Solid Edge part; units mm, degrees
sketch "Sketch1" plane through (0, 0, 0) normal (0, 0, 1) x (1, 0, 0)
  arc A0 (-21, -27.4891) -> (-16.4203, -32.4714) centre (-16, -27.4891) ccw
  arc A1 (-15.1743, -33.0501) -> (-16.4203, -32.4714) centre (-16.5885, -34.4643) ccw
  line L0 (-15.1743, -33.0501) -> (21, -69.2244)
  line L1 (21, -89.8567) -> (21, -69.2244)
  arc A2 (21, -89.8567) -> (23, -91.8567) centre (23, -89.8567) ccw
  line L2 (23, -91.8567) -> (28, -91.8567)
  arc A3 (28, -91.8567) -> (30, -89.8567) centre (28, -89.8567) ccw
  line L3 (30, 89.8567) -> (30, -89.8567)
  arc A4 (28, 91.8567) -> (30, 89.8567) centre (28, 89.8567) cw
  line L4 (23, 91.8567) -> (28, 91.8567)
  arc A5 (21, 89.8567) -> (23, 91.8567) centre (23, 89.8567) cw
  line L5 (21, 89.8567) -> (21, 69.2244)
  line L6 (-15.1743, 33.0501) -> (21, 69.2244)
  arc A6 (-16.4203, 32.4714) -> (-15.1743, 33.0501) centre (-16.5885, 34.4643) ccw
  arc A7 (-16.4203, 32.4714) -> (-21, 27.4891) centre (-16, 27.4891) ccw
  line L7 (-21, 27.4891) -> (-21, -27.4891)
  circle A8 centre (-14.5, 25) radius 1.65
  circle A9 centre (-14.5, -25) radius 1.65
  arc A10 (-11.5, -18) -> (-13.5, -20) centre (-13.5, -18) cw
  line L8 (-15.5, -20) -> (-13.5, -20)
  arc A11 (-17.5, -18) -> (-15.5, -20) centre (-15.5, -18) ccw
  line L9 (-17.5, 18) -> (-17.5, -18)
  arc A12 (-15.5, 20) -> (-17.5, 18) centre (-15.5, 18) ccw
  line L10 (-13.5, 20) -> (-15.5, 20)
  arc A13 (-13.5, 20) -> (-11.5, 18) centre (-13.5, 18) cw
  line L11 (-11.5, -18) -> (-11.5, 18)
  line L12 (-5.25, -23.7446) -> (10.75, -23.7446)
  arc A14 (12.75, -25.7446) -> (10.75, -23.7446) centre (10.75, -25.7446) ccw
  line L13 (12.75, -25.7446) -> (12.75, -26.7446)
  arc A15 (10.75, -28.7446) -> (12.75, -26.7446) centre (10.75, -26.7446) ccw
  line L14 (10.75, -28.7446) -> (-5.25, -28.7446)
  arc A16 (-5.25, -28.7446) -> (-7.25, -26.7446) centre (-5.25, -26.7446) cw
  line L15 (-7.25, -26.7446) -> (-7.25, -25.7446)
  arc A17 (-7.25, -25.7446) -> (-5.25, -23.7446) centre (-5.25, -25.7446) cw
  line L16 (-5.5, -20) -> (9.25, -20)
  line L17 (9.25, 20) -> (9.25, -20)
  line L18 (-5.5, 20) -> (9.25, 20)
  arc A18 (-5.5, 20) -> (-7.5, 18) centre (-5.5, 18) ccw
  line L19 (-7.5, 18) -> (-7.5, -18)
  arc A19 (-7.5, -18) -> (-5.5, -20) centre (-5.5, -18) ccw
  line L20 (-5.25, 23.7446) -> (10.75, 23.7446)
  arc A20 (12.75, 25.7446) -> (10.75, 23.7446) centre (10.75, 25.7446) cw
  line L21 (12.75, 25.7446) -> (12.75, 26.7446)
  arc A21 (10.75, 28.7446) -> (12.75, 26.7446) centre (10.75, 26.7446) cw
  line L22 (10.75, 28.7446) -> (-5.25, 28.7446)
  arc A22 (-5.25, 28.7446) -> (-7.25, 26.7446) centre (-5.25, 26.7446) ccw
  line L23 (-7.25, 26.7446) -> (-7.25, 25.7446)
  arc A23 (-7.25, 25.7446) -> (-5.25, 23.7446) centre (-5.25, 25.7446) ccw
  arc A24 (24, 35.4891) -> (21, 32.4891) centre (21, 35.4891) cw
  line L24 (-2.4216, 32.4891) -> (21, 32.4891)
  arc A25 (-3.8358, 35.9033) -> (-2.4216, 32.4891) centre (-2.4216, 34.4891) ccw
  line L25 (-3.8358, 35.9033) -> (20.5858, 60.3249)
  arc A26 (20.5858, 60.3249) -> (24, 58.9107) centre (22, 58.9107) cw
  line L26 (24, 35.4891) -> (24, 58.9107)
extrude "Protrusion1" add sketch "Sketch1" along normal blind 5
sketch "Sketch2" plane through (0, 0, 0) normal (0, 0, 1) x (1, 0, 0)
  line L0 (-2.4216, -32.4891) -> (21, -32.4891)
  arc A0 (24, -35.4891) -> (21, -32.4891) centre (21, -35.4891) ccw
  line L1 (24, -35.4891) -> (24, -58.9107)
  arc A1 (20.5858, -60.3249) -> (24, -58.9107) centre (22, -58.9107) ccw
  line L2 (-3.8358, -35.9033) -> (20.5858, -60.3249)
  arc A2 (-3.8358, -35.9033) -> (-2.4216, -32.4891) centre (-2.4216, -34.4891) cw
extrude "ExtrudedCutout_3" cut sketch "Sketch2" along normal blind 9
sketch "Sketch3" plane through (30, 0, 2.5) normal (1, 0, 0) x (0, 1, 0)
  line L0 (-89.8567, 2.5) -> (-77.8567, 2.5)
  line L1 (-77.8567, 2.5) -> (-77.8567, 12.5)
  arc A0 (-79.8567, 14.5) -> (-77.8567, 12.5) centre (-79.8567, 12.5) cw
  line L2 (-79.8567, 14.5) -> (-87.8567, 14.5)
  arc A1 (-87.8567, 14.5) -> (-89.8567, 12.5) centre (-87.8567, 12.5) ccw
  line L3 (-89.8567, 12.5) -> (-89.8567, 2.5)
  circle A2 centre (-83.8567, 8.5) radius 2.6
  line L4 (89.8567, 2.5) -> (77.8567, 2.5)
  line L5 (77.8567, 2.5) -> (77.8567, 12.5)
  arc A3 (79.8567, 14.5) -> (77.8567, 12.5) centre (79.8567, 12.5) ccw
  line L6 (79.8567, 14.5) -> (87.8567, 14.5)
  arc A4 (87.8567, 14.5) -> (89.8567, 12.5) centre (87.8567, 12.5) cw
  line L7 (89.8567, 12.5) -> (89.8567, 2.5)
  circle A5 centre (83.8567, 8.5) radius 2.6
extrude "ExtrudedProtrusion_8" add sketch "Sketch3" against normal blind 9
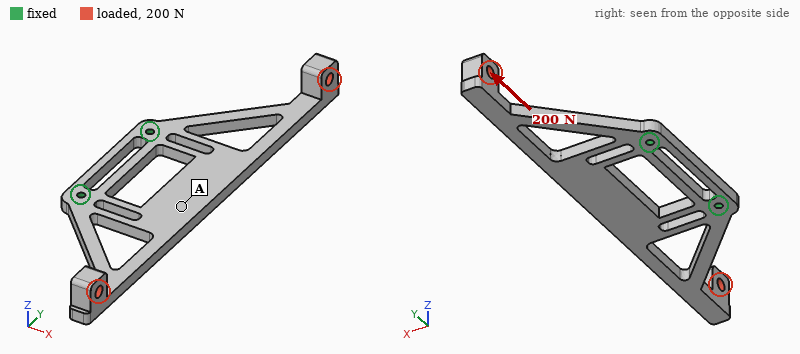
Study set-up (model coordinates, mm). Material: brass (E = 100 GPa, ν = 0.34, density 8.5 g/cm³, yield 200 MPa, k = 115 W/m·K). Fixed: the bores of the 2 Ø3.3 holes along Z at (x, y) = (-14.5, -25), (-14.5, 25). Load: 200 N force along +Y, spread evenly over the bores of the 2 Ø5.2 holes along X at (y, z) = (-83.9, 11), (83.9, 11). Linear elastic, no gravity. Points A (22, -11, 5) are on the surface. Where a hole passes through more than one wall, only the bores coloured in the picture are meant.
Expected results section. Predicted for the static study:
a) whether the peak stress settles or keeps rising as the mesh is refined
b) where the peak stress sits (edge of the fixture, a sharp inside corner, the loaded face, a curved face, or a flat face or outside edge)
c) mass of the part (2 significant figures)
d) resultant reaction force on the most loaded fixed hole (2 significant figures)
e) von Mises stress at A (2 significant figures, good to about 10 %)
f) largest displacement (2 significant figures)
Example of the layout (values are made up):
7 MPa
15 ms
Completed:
keeps rising
edge of the fixture
170 g
150 N
4.7 MPa
0.19 mm
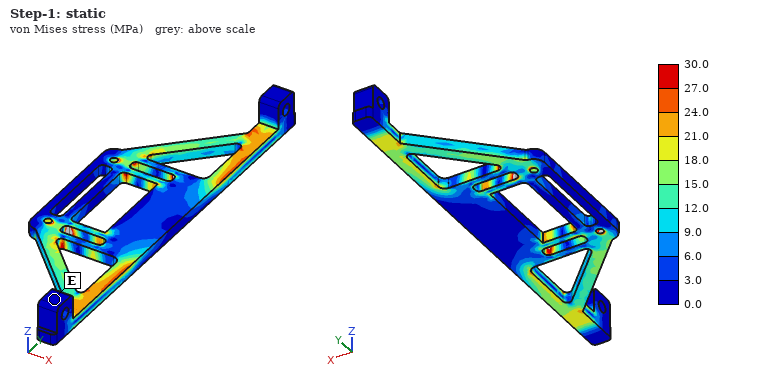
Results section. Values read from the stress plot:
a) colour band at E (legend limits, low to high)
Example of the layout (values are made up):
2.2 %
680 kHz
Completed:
0.0 to 3.0 MPa
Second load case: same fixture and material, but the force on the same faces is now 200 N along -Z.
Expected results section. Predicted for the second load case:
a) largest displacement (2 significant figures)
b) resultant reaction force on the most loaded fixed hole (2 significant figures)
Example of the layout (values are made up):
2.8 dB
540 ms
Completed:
0.95 mm
100 N
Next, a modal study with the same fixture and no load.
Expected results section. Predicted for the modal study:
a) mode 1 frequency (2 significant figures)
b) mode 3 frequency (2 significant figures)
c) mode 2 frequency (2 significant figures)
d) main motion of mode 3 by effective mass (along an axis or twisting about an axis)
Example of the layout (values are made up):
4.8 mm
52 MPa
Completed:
380 Hz
790 Hz
390 Hz
along Z
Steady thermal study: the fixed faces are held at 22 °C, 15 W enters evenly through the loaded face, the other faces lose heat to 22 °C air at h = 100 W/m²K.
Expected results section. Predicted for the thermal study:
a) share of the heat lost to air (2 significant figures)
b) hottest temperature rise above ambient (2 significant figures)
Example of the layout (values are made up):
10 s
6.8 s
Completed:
82 %
36 K
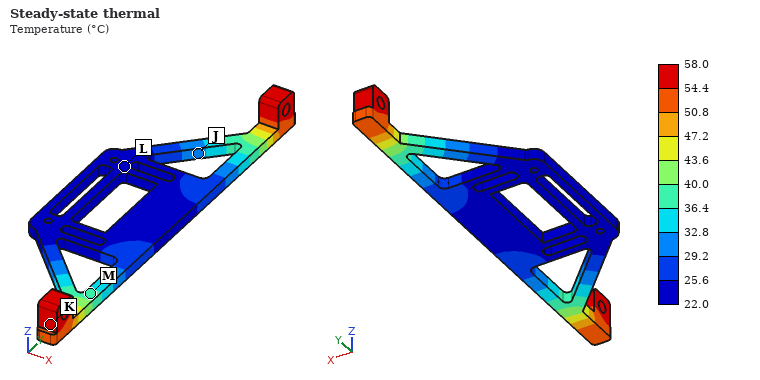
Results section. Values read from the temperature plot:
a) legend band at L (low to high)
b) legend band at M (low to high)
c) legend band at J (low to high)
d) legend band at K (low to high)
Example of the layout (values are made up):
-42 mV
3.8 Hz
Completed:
22.0 to 25.6 °C
36.4 to 40.0 °C
29.2 to 32.8 °C
54.4 to 58.0 °C
